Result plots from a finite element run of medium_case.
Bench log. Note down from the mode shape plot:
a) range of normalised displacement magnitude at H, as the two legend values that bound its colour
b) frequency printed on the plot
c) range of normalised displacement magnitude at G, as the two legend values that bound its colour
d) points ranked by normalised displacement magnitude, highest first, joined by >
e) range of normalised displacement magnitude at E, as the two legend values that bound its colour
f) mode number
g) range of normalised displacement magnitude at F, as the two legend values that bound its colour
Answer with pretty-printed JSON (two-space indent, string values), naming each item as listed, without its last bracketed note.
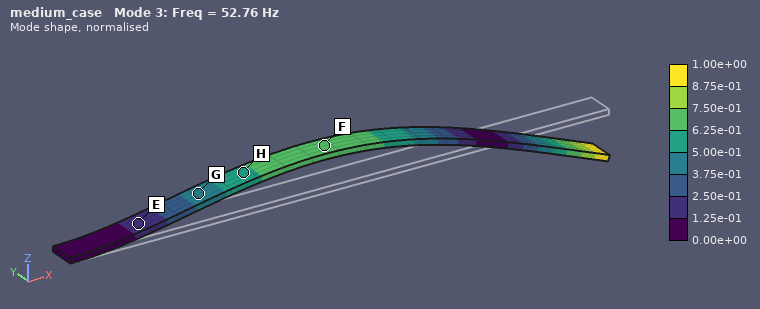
{
  "range of normalised displacement magnitude at H, as the two legend values that bound its colour": "5.00e-01 to 6.25e-01",
  "frequency printed on the plot": "52.76 Hz",
  "range of normalised displacement magnitude at G, as the two legend values that bound its colour": "3.75e-01 to 5.00e-01",
  "points ranked by normalised displacement magnitude, highest first, joined by >": "F > H > G > E",
  "range of normalised displacement magnitude at E, as the two legend values that bound its colour": "1.25e-01 to 2.50e-01",
  "mode number": "3",
  "range of normalised displacement magnitude at F, as the two legend values that bound its colour": "6.25e-01 to 7.50e-01"
}
